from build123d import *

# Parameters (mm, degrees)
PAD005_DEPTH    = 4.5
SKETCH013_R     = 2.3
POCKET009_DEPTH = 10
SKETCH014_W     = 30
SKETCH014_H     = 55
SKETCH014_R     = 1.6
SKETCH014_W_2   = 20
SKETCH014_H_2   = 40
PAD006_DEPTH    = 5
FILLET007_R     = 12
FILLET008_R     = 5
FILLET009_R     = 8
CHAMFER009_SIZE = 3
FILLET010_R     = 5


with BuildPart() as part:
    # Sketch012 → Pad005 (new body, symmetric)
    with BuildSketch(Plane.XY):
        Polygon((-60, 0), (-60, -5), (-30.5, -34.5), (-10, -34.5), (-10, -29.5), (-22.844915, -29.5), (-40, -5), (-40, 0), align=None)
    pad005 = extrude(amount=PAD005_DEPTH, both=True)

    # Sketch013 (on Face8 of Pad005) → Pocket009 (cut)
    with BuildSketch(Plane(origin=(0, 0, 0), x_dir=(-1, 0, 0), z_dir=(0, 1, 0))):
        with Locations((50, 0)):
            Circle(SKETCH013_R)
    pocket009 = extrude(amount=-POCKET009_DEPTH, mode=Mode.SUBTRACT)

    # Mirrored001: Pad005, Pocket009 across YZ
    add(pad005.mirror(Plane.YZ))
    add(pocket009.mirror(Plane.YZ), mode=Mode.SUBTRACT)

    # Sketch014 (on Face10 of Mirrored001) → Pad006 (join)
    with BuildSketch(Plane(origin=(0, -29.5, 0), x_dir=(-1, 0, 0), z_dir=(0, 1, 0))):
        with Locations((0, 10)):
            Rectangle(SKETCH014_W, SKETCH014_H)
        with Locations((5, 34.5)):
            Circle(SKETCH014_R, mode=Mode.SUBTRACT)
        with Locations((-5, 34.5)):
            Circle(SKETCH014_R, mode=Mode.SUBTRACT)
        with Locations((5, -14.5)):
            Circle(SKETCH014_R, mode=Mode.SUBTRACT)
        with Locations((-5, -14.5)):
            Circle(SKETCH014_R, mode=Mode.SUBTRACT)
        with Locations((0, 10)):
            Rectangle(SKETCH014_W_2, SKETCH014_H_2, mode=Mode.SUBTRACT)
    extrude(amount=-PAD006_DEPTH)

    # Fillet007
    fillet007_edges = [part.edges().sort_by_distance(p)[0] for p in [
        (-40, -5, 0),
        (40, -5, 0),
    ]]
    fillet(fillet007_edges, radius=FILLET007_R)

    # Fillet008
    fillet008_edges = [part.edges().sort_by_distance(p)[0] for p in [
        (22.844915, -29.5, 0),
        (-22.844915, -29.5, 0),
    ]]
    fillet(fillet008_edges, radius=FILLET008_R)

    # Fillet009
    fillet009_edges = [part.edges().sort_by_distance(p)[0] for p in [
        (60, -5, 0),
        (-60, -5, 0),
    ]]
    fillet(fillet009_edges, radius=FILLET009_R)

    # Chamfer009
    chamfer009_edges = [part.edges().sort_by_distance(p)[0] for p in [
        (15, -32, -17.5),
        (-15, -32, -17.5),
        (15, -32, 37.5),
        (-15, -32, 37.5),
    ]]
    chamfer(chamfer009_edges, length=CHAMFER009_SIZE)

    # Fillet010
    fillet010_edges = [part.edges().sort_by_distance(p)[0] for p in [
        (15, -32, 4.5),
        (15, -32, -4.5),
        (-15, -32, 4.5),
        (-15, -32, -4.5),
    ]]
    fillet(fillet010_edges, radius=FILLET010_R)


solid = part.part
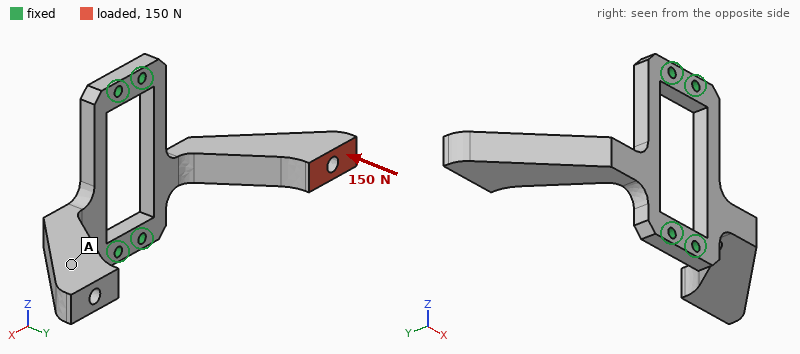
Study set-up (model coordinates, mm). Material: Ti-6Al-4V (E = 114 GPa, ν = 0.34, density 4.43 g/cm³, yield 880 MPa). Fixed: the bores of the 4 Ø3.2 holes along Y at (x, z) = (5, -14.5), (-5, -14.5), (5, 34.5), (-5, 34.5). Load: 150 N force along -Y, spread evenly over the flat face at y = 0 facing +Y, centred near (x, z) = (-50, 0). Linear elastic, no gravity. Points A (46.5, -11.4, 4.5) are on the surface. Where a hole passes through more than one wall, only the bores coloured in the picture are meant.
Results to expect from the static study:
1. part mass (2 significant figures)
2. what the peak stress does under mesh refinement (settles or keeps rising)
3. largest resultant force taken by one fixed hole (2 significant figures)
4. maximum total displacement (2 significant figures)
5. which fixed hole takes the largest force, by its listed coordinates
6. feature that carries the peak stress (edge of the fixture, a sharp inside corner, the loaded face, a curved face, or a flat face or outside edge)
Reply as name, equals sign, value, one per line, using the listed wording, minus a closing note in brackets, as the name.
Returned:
part mass = 64 g
what the peak stress does under mesh refinement = keeps rising
largest resultant force taken by one fixed hole = 170 N
maximum total displacement = 0.86 mm
which fixed hole takes the largest force, by its listed coordinates = (-5, -14.5)
feature that carries the peak stress = a sharp inside corner
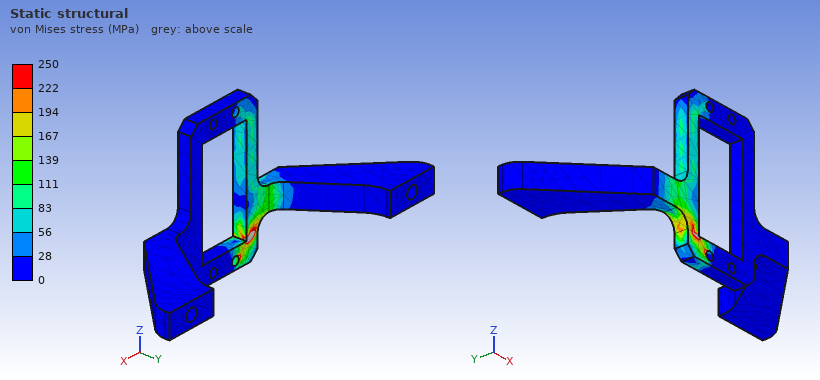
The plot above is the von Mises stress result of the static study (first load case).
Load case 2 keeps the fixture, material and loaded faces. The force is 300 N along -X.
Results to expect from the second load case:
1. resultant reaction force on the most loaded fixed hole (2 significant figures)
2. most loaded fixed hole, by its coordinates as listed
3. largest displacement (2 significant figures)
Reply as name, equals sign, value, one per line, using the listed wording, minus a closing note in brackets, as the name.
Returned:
resultant reaction force on the most loaded fixed hole = 240 N
most loaded fixed hole, by its coordinates as listed = (-5, -14.5)
largest displacement = 1.5 mm
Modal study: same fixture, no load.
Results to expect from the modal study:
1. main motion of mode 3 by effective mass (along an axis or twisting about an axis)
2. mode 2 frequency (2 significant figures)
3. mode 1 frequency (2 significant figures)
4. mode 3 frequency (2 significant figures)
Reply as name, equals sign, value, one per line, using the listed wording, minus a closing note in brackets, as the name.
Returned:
main motion of mode 3 by effective mass = along Z
mode 2 frequency = 600 Hz
mode 1 frequency = 600 Hz
mode 3 frequency = 1100 Hz
